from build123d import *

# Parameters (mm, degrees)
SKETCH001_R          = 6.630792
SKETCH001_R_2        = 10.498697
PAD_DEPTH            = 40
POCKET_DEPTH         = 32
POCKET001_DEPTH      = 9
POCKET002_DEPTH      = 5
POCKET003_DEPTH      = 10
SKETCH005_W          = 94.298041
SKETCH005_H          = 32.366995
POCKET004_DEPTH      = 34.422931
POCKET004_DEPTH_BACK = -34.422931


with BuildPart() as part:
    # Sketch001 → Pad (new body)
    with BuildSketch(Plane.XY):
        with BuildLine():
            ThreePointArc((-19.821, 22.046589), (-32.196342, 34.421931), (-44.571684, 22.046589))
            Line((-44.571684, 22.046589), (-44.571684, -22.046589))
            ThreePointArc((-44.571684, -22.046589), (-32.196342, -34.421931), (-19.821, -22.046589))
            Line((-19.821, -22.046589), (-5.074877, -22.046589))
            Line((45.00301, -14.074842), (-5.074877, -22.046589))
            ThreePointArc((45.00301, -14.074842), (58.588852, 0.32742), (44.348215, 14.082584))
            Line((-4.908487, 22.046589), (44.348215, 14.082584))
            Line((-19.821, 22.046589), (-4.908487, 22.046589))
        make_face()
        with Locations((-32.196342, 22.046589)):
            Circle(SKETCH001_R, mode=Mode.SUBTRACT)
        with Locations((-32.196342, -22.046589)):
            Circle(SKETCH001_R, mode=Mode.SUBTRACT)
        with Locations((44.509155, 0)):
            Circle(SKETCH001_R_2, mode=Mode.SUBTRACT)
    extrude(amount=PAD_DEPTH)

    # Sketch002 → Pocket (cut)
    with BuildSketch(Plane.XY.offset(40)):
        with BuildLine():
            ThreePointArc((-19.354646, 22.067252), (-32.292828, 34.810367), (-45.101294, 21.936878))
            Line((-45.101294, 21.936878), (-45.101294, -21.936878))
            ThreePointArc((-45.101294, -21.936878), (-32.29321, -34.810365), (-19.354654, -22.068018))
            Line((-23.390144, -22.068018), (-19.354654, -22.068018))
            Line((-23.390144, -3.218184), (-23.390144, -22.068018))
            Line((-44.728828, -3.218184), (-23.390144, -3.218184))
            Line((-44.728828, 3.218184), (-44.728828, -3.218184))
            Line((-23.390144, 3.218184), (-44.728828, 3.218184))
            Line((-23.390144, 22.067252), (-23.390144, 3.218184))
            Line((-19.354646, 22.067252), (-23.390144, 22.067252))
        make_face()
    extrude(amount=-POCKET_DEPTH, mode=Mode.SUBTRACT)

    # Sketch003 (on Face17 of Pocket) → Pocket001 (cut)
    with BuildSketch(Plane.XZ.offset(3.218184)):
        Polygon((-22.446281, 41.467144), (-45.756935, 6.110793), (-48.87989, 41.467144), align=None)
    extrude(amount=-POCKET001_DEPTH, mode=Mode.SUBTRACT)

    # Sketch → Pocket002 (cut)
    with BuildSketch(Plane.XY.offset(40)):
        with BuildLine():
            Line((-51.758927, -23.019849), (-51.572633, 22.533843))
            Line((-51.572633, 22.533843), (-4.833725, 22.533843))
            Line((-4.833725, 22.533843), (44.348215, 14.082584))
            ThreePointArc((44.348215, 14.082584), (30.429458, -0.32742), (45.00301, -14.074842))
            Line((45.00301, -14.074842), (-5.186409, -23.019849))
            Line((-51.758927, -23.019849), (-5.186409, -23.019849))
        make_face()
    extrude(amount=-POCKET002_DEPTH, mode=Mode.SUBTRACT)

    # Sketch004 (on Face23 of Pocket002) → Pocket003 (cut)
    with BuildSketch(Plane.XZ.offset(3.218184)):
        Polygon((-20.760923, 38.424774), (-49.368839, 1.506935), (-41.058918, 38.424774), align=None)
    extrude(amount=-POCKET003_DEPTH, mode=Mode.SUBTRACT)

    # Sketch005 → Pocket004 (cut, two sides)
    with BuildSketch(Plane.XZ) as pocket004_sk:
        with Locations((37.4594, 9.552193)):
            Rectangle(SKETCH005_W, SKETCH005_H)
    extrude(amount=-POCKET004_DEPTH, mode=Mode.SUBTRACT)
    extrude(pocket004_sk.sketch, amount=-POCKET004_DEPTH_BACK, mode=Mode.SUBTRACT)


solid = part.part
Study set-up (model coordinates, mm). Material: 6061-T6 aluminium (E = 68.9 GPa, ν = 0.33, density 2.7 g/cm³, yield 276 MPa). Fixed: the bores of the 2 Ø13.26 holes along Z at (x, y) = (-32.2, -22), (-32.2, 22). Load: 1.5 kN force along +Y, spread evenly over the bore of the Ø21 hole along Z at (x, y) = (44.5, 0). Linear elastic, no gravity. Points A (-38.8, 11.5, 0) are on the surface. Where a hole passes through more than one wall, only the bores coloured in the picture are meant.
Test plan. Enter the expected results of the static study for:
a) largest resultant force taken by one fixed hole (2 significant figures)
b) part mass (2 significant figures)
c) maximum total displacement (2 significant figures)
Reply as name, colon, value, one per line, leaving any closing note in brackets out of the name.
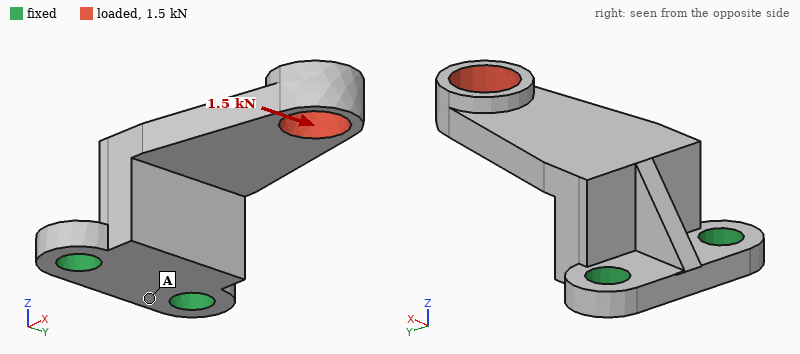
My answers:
largest resultant force taken by one fixed hole: 2.9 kN
part mass: 140 g
maximum total displacement: 0.23 mm
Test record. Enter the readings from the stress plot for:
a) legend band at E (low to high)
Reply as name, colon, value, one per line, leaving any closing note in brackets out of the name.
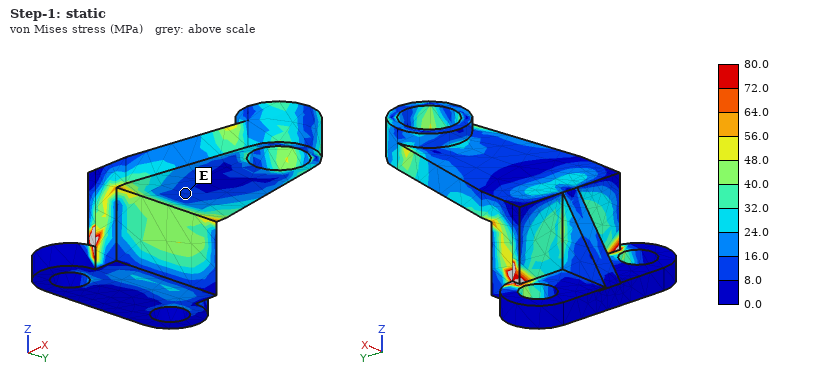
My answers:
legend band at E: 8.0 to 16.0 MPa
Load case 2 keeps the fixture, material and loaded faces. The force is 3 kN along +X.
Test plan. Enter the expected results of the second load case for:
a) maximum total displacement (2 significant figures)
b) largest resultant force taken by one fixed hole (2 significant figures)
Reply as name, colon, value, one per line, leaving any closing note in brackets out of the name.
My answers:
maximum total displacement: 0.46 mm
largest resultant force taken by one fixed hole: 1.5 kN
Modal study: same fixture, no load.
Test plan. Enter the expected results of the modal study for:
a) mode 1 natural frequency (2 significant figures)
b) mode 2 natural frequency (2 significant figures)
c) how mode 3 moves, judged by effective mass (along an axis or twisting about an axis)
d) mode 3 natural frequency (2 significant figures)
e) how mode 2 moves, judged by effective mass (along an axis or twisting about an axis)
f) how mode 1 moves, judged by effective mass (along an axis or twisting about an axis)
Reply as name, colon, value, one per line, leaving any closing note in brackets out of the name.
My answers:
mode 1 natural frequency: 1400 Hz
mode 2 natural frequency: 3200 Hz
how mode 3 moves, judged by effective mass: along X
mode 3 natural frequency: 4100 Hz
how mode 2 moves, judged by effective mass: along Y
how mode 1 moves, judged by effective mass: along Z
